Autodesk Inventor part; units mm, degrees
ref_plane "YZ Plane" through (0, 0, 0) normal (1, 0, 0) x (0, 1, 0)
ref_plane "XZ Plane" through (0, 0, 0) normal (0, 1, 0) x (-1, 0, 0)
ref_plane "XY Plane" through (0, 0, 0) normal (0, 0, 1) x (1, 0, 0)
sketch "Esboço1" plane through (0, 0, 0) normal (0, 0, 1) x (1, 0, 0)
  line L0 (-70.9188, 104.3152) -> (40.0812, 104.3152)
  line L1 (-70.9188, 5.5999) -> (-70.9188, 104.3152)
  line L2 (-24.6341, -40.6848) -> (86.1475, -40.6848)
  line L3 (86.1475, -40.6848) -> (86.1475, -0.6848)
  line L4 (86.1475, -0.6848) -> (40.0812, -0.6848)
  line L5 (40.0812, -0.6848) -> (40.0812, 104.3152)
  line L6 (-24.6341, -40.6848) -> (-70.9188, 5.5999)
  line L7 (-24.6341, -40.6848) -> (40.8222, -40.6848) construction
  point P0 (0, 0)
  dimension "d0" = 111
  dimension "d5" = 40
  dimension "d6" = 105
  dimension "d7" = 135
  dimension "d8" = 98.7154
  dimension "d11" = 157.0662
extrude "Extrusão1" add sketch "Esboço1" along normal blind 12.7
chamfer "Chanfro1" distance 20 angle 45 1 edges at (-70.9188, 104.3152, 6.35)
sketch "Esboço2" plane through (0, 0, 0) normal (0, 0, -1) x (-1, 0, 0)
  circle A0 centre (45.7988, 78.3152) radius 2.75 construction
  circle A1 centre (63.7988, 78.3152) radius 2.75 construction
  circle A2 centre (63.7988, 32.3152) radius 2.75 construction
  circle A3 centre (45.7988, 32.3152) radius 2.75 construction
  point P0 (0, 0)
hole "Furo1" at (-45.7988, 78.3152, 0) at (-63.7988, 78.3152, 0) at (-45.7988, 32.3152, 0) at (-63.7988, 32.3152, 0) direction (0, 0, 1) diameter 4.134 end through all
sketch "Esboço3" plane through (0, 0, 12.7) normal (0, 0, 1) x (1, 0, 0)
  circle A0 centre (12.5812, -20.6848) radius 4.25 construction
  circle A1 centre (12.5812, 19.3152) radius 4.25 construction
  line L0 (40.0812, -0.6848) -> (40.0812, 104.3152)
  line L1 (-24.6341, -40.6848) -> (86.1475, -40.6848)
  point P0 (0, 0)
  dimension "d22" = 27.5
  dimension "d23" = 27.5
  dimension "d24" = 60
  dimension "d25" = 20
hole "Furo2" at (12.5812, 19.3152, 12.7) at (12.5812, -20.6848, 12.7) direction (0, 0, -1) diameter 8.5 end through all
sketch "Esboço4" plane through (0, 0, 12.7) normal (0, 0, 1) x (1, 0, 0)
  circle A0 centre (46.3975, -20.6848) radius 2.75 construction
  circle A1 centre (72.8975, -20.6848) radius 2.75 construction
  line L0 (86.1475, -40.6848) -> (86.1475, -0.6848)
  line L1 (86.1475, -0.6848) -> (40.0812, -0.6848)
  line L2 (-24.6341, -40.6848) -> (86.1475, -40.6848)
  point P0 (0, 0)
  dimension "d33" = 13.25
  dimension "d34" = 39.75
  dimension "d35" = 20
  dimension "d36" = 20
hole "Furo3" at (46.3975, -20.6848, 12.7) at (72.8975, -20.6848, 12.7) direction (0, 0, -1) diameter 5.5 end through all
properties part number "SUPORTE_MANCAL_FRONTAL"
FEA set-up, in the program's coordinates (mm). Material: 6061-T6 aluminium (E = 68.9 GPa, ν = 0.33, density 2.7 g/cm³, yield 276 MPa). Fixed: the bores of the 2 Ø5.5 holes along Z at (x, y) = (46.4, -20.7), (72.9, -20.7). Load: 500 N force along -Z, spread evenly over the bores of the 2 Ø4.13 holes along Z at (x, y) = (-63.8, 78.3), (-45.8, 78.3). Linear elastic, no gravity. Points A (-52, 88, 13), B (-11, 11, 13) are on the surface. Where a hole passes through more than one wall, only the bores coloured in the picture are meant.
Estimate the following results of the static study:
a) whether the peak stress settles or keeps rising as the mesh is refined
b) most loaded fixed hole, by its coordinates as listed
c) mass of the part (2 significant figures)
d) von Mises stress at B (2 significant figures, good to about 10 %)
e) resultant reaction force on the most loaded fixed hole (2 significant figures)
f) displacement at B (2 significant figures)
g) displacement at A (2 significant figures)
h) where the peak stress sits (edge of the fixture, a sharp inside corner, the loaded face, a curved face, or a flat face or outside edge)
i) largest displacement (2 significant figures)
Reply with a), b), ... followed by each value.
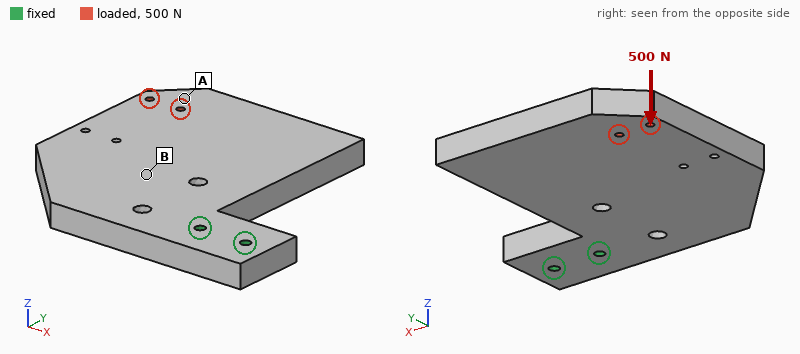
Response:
a) keeps rising
b) (46.4, -20.7)
c) 560 g
d) 15 MPa
e) 1.3 kN
f) 0.25 mm
g) 0.82 mm
h) edge of the fixture
i) 0.90 mm
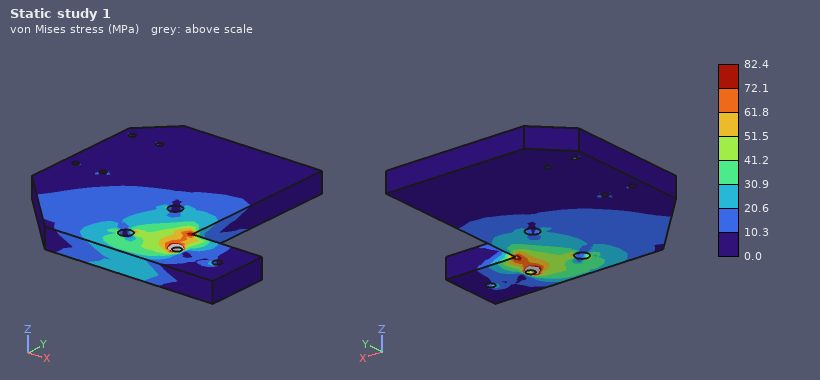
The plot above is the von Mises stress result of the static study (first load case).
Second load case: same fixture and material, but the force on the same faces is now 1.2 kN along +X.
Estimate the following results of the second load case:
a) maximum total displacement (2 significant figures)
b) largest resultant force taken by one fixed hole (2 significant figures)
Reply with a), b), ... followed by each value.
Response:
a) 0.20 mm
b) 3.7 kN
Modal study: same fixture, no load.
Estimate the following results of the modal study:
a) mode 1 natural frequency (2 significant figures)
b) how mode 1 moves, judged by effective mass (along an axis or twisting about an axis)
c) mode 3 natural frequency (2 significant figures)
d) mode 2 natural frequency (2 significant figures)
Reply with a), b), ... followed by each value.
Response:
a) 310 Hz
b) along Z
c) 750 Hz
d) 730 Hz
